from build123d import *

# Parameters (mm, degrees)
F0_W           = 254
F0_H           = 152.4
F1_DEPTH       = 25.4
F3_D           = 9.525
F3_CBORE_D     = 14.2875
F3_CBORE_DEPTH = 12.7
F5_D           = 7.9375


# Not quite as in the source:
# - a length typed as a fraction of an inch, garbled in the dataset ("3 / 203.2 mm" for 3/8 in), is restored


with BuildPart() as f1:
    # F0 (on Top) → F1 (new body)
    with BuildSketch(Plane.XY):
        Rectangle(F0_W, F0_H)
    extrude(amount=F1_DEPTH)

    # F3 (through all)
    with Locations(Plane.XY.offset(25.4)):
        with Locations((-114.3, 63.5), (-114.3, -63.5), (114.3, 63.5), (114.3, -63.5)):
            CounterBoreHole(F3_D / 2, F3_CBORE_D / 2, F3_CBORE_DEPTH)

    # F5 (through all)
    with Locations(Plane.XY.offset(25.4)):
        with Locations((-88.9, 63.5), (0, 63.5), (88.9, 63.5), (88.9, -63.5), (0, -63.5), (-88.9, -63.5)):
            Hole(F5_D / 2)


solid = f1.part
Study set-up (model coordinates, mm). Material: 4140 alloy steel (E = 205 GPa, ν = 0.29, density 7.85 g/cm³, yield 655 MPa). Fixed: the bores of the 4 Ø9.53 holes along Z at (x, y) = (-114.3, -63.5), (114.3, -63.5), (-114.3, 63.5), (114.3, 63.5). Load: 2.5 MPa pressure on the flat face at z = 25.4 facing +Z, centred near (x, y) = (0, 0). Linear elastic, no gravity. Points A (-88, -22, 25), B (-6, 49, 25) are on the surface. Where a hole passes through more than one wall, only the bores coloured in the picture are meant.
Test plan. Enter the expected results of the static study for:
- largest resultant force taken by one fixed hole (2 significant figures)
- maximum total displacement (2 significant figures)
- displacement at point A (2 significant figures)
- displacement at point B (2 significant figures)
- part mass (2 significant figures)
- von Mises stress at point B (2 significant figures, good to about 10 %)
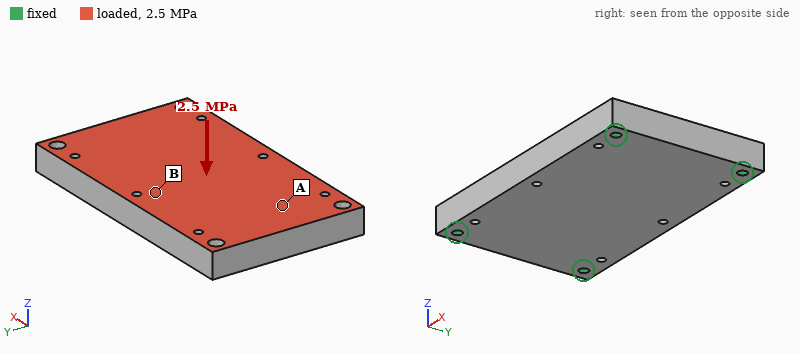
32 kN
0.17 mm
0.072 mm
0.16 mm
7.6 kg
97 MPa
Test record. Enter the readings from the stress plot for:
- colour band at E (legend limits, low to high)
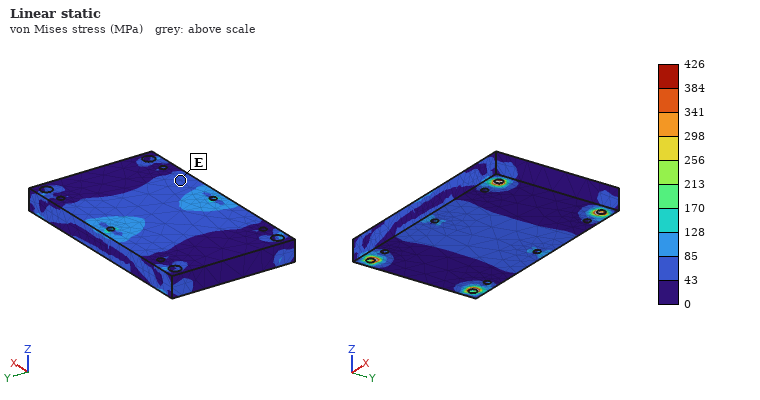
43 to 85 MPa
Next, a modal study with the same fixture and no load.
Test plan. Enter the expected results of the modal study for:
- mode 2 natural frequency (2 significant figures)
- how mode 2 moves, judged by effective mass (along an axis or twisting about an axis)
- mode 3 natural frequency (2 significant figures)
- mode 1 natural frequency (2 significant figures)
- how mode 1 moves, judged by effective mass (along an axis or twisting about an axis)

2800 Hz
twisting about X
4000 Hz
1500 Hz
along Z
